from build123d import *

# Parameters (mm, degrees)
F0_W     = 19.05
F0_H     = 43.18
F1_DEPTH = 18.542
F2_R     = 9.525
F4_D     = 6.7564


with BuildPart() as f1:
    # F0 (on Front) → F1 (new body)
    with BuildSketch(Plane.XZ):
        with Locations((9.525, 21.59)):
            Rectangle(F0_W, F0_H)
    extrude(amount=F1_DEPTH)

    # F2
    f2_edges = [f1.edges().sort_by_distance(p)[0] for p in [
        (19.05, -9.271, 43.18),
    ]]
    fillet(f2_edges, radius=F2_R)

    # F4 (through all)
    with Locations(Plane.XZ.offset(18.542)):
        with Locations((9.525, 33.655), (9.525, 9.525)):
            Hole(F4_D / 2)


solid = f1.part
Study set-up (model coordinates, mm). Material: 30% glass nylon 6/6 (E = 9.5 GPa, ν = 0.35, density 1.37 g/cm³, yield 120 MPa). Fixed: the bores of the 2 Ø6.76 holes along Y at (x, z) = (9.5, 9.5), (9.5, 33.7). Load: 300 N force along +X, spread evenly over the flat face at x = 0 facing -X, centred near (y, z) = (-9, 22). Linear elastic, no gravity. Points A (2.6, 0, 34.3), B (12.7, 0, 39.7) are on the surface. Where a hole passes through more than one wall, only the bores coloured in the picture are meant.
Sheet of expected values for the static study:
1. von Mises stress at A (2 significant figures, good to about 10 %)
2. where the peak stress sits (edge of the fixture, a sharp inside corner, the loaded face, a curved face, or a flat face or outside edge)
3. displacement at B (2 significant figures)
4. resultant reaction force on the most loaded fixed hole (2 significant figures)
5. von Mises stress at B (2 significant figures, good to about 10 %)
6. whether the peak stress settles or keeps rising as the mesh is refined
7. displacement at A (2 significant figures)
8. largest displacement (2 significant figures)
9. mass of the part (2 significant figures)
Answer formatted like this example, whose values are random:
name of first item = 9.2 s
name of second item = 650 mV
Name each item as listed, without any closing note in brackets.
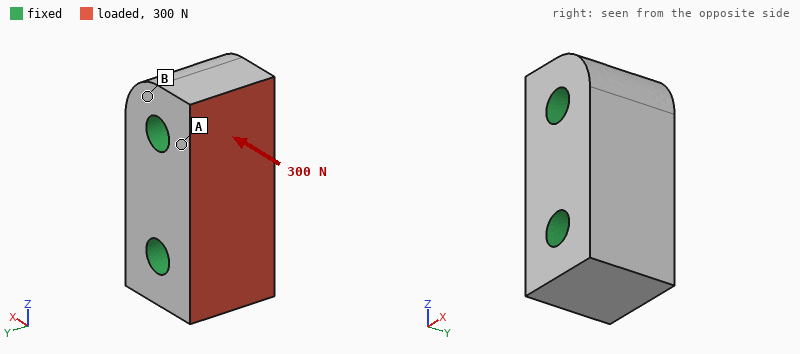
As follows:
von Mises stress at A = 0.44 MPa
where the peak stress sits = edge of the fixture
displacement at B = 0.16 µm
resultant reaction force on the most loaded fixed hole = 150 N
von Mises stress at B = 0.21 MPa
whether the peak stress settles or keeps rising as the mesh is refined = keeps rising
displacement at A = 0.24 µm
largest displacement = 0.74 µm
mass of the part = 19 g
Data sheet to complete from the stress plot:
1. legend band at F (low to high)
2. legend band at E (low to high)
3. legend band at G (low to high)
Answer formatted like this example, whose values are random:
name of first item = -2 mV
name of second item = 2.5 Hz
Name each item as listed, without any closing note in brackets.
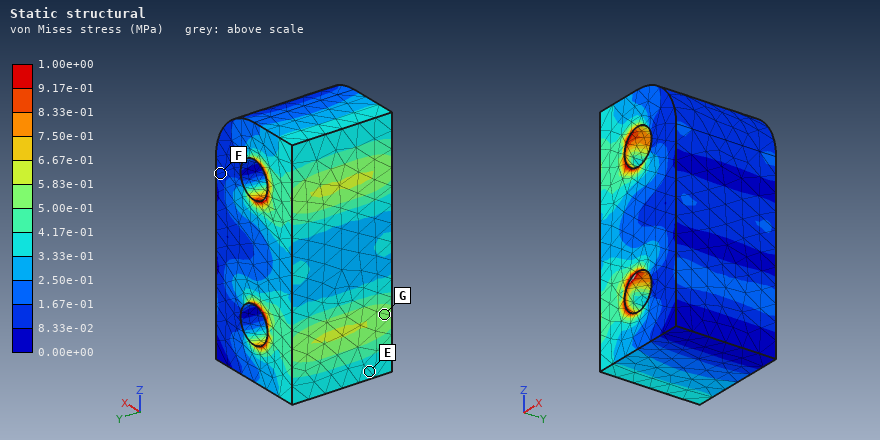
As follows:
legend band at F = 8.33e-02 to 1.67e-01 MPa
legend band at E = 3.33e-01 to 4.17e-01 MPa
legend band at G = 5.00e-01 to 5.83e-01 MPa
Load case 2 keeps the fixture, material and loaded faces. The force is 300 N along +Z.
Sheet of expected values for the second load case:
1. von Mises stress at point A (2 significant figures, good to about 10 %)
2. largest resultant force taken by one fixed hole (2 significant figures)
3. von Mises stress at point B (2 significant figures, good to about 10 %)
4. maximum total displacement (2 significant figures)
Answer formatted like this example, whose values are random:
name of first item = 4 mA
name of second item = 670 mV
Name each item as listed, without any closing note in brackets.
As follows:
von Mises stress at point A = 0.77 MPa
largest resultant force taken by one fixed hole = 170 N
von Mises stress at point B = 0.33 MPa
maximum total displacement = 2.1 µm
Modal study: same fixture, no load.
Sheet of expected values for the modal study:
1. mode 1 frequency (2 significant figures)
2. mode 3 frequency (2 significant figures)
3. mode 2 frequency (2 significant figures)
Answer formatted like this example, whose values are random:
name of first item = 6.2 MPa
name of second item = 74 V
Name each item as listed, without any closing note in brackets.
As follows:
mode 1 frequency = 29 kHz
mode 3 frequency = 32 kHz
mode 2 frequency = 32 kHz
